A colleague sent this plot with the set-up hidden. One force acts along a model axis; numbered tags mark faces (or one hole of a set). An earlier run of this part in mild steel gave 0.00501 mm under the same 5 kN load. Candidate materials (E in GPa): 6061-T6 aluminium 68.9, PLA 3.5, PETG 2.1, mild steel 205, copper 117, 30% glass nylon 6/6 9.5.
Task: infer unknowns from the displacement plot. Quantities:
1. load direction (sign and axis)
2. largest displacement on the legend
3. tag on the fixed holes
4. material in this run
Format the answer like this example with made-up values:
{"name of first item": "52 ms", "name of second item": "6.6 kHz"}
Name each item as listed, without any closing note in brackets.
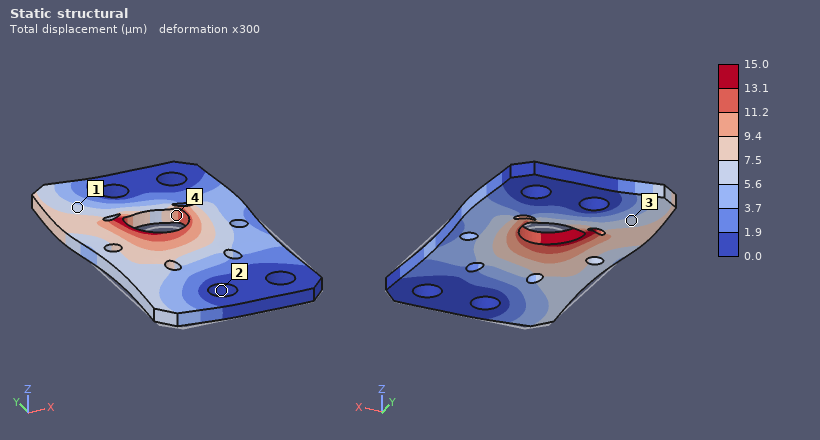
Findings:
{"load direction": "+Y", "largest displacement on the legend": "15.0 µm", "tag on the fixed holes": "2", "material in this run": "6061-T6 aluminium"}
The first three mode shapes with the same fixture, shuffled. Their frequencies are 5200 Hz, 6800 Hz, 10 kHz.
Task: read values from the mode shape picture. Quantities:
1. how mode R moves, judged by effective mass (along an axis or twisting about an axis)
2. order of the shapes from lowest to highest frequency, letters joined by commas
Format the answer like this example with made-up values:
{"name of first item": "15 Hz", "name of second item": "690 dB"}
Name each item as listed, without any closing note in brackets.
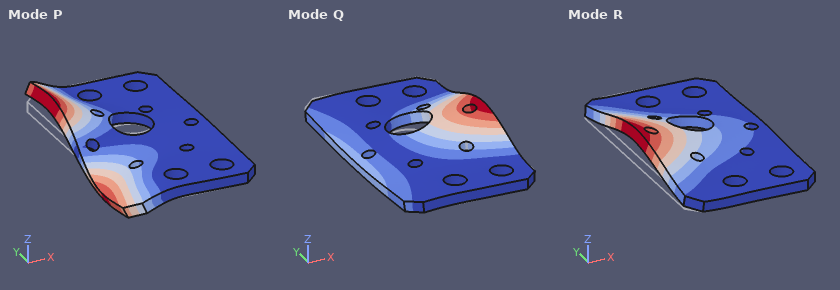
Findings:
{"how mode R moves, judged by effective mass": "along Z", "order of the shapes from lowest to highest frequency, letters joined by commas": "R, Q, P"}
